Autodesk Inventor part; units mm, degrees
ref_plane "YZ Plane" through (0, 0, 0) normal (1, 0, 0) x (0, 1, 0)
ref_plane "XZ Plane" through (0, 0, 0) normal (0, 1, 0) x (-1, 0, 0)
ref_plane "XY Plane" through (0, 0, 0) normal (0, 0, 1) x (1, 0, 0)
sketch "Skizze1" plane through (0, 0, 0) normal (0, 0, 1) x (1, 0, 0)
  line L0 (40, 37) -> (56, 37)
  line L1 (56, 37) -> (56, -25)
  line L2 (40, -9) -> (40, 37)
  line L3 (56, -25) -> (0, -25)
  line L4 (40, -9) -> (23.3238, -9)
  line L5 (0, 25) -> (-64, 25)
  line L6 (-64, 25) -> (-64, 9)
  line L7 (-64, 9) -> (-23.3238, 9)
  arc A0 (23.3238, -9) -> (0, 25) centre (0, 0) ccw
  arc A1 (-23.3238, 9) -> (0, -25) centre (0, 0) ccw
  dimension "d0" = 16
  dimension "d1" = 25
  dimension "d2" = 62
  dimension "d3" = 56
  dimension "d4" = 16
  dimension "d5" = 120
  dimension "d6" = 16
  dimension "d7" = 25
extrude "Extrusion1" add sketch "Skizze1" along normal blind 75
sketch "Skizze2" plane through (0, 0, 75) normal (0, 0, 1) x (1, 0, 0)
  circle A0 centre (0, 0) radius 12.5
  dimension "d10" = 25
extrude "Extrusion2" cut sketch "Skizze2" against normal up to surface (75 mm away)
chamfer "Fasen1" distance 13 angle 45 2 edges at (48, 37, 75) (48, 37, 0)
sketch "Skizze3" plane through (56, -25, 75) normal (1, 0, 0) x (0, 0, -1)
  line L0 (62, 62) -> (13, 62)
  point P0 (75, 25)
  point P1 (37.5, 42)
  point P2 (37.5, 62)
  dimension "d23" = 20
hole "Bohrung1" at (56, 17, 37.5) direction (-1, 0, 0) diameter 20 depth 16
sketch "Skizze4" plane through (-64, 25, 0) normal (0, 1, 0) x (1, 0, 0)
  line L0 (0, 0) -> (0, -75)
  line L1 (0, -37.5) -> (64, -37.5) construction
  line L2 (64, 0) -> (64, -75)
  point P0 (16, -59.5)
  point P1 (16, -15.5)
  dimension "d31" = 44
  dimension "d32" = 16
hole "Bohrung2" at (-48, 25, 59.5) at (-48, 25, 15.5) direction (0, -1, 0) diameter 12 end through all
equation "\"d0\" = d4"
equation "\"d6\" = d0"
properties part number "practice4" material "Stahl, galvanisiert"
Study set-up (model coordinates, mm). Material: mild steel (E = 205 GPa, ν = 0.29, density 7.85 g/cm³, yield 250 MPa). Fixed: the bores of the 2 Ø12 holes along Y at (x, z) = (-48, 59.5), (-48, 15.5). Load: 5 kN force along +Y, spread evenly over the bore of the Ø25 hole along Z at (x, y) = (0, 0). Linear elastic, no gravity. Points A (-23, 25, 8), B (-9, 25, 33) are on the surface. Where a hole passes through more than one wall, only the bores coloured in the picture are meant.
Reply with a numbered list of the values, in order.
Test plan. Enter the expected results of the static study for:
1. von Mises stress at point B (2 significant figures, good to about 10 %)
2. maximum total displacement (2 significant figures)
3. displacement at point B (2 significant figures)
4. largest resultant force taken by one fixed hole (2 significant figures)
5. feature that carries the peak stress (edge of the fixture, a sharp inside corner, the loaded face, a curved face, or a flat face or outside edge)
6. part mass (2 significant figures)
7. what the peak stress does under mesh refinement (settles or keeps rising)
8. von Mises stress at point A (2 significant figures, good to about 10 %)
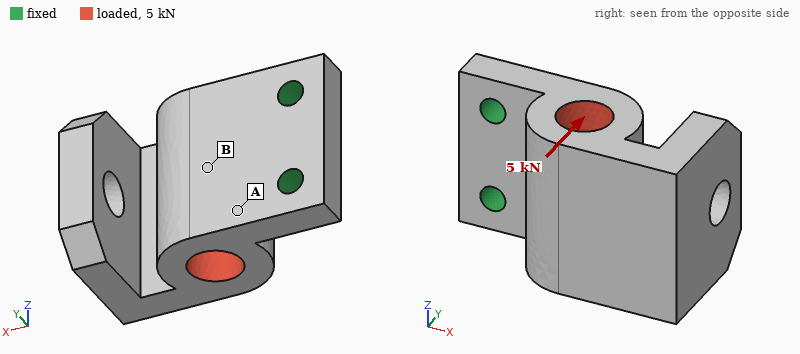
1. 13 MPa
2. 95 µm
3. 26 µm
4. 2.5 kN
5. edge of the fixture
6. 2.0 kg
7. keeps rising
8. 32 MPa
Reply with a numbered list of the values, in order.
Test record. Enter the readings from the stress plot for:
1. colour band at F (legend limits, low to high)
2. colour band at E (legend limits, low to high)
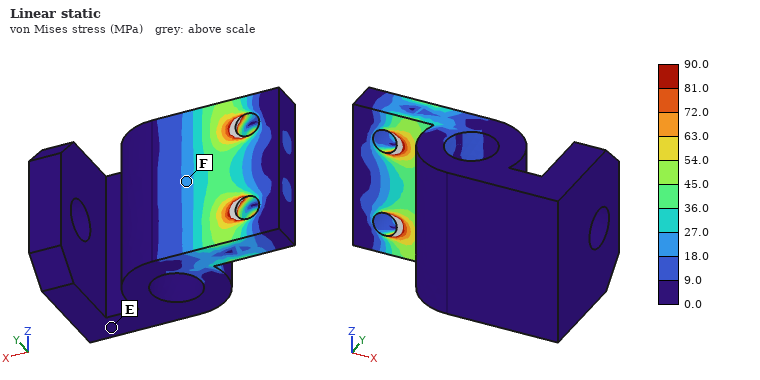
1. 18.0 to 27.0 MPa
2. 0.0 to 9.0 MPa
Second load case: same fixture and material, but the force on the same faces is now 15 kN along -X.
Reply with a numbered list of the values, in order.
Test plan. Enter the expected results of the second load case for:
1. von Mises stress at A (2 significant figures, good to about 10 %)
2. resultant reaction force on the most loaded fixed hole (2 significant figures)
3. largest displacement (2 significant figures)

1. 52 MPa
2. 7.6 kN
3. 0.15 mm
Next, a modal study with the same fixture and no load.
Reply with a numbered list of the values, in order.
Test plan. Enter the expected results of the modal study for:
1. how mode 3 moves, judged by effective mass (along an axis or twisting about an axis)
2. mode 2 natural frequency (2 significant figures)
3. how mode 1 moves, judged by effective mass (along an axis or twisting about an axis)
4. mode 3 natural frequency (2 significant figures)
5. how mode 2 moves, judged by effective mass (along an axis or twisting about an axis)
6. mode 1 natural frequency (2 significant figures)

1. along X
2. 2300 Hz
3. along Y
4. 2600 Hz
5. along Z
6. 800 Hz
